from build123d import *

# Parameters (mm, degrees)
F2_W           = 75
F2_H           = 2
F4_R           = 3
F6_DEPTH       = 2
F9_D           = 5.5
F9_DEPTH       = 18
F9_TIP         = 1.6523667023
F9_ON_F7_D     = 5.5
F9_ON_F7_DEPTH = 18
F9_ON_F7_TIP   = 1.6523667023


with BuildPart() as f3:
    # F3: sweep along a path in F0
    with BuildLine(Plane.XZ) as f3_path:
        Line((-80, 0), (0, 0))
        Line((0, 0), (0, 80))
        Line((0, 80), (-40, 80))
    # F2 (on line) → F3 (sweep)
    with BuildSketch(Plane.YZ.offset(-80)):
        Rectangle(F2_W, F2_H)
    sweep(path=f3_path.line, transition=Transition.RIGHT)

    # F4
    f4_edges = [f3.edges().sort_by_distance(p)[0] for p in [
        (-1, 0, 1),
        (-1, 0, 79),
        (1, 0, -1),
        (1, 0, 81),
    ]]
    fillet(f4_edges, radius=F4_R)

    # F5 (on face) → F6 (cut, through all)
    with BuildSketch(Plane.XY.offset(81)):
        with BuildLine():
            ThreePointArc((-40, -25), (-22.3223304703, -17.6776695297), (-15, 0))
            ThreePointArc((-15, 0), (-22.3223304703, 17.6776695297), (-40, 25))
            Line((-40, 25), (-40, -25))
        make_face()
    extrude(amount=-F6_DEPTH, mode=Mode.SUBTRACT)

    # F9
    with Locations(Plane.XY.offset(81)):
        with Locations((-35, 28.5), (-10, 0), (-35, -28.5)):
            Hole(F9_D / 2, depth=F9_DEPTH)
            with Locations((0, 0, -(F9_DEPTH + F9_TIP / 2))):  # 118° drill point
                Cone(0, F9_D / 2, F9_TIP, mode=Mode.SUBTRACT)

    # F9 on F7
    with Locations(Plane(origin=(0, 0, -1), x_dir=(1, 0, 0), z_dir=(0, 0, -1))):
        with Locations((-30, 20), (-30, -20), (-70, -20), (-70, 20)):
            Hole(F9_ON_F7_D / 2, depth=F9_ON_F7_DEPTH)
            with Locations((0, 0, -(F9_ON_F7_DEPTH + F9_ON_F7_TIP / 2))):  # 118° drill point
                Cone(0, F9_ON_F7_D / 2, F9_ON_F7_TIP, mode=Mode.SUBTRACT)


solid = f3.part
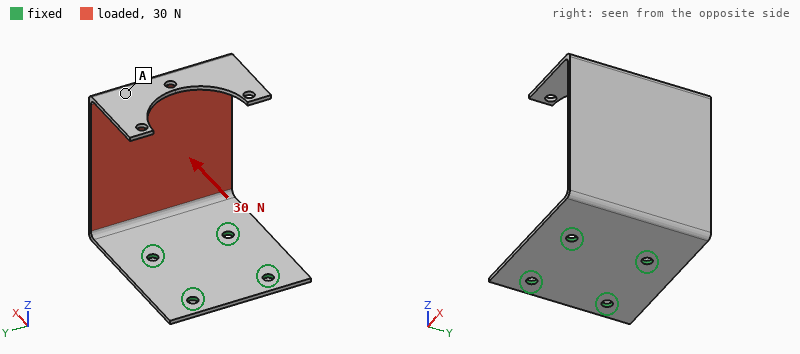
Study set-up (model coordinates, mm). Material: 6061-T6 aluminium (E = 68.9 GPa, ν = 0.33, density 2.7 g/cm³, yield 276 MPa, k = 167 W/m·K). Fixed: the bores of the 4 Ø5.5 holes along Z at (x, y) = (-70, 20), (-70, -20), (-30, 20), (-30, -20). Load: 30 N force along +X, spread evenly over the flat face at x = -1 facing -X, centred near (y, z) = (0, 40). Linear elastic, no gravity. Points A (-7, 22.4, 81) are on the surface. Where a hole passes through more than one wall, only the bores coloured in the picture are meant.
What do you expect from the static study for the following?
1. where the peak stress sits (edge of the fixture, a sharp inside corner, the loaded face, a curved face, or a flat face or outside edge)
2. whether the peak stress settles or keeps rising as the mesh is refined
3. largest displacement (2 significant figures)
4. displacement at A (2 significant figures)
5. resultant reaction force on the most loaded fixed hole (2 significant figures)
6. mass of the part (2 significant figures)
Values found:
edge of the fixture
keeps rising
1.3 mm
1.2 mm
13 N
75 g
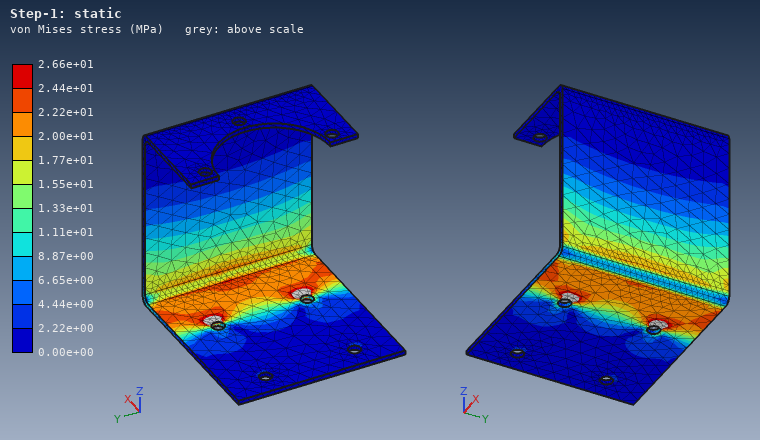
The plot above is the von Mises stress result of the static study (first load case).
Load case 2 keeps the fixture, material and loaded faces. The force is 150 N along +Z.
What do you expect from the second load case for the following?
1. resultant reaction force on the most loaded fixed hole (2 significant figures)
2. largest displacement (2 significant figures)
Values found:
85 N
1.3 mm
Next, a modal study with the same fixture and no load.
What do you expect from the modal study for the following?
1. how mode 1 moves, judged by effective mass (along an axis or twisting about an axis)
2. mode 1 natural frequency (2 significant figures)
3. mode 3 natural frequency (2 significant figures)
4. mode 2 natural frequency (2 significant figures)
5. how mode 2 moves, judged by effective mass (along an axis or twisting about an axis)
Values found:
along X
120 Hz
460 Hz
260 Hz
along Y
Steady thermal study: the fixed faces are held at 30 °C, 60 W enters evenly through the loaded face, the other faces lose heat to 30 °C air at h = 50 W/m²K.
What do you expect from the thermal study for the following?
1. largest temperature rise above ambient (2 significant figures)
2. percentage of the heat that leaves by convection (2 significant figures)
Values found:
66 K
60 %
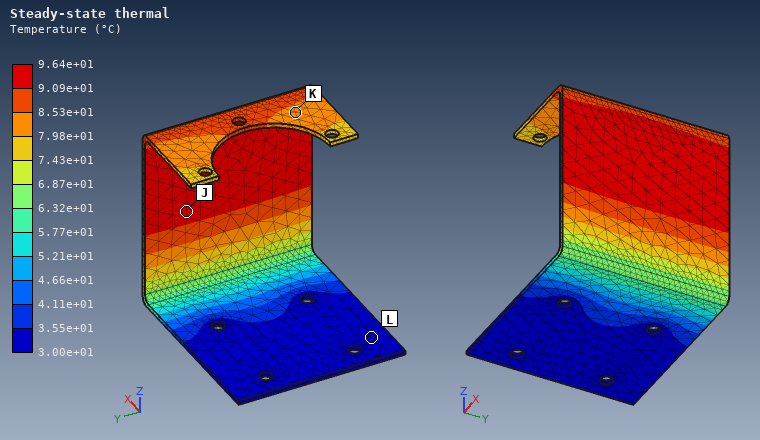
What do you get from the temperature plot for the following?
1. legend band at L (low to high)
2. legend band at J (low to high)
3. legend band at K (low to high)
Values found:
3.00e+01 to 3.55e+01 °C
9.09e+01 to 9.64e+01 °C
7.98e+01 to 8.53e+01 °C
